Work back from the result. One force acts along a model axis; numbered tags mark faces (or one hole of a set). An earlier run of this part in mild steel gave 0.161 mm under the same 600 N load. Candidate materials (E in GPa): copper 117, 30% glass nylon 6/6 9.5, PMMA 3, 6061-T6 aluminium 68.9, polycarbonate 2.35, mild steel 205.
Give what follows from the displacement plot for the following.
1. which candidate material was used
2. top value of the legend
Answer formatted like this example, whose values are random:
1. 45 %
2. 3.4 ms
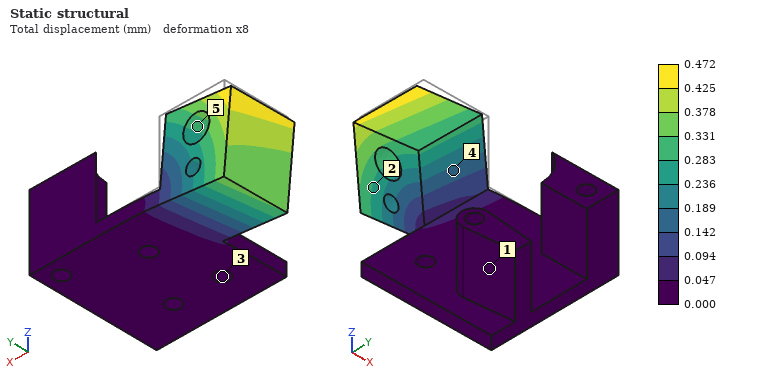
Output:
1. 6061-T6 aluminium
2. 0.472 mm
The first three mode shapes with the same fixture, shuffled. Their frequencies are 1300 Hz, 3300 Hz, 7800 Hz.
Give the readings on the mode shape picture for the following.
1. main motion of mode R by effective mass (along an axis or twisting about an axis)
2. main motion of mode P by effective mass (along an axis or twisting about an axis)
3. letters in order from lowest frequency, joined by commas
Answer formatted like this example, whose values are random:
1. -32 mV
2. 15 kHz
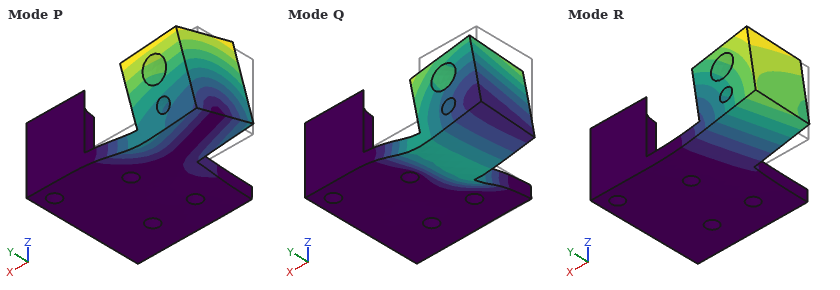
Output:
1. along Z
2. along Y
3. R, P, Q
